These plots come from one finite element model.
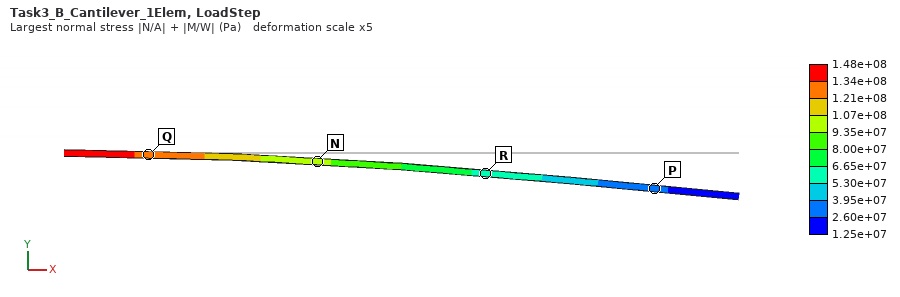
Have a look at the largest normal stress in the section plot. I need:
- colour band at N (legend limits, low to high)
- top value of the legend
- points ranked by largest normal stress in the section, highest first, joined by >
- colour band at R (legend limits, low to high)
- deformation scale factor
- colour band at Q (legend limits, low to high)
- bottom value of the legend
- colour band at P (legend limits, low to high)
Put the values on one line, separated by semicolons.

9.35e+07 to 1.07e+08 Pa; 1.48e+08 Pa; Q > N > R > P; 5.30e+07 to 6.65e+07 Pa; 5; 1.21e+08 to 1.34e+08 Pa; 1.25e+07 Pa; 2.60e+07 to 3.95e+07 Pa
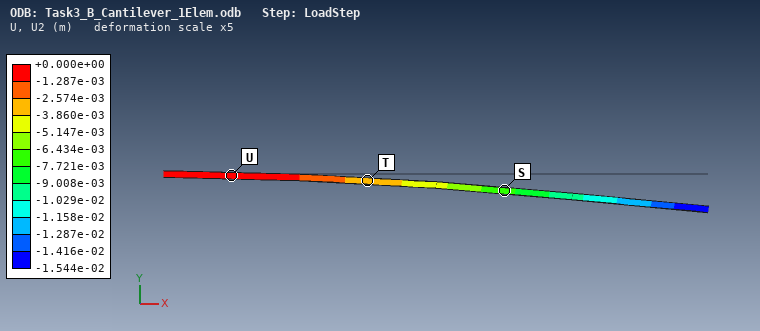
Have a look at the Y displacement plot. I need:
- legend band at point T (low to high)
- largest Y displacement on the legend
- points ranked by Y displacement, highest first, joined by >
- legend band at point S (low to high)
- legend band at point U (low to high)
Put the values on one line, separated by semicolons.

-3.860e-03 to -2.574e-03 m; +0.000e+00 m; U > T > S; -7.721e-03 to -6.434e-03 m; -1.287e-03 to +0.000e+00 m
